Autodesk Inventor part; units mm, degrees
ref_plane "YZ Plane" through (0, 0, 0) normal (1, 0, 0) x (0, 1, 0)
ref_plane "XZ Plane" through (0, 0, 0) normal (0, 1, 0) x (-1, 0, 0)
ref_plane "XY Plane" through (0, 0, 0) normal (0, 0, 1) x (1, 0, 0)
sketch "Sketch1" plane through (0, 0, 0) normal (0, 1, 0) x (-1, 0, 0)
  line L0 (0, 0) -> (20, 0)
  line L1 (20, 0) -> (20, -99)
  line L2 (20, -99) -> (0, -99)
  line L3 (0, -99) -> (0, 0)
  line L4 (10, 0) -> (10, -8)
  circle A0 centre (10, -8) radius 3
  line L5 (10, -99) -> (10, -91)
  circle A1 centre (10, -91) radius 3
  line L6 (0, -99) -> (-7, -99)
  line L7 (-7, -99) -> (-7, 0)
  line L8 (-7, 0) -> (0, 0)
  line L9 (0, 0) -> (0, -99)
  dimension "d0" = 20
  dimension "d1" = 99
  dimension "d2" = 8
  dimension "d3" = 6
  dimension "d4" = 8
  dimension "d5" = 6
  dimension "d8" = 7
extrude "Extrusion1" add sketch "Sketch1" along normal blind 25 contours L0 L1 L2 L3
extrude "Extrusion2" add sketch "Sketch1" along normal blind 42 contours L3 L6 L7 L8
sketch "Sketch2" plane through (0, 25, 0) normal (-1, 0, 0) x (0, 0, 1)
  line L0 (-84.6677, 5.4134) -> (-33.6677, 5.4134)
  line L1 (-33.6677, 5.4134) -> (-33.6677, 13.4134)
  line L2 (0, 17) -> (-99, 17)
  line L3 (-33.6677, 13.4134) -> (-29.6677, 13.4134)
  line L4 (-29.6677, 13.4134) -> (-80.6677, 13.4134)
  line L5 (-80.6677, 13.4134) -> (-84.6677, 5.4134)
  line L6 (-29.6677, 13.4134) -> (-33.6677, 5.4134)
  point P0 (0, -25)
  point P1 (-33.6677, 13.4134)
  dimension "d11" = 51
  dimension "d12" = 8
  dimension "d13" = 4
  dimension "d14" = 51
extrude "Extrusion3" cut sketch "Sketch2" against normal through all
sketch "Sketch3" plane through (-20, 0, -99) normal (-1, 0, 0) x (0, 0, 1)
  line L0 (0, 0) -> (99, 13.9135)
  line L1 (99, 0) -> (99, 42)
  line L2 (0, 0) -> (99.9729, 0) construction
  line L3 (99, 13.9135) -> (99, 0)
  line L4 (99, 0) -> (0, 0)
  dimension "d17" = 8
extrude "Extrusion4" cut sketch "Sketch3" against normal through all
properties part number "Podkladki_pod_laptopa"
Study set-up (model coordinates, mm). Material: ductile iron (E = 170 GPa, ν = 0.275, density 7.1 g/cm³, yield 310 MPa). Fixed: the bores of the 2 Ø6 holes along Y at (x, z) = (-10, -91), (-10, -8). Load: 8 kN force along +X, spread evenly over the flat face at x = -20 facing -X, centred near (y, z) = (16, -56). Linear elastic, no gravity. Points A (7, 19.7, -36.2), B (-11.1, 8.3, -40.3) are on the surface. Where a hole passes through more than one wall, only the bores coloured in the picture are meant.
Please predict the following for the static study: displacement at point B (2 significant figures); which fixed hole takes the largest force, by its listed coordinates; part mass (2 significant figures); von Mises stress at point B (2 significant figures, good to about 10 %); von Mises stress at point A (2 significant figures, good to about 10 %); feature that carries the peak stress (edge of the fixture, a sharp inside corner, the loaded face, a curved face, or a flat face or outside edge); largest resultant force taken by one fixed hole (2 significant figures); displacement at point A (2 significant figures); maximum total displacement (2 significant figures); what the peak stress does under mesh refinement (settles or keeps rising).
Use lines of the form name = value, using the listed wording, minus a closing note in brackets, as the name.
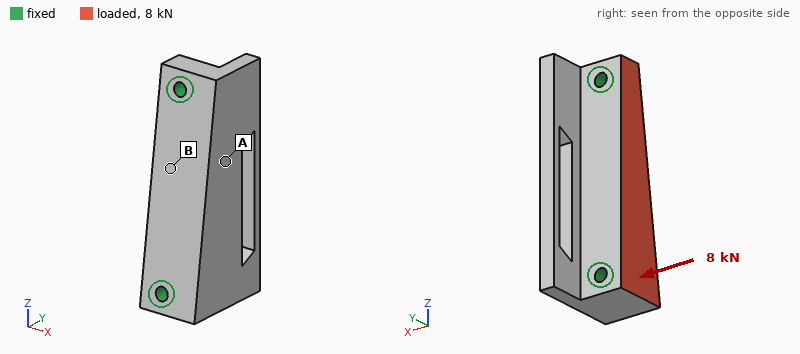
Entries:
displacement at point B = 6.7 µm
which fixed hole takes the largest force, by its listed coordinates = (-10, -91)
part mass = 400 g
von Mises stress at point B = 5.2 MPa
von Mises stress at point A = 17 MPa
feature that carries the peak stress = edge of the fixture
largest resultant force taken by one fixed hole = 4.8 kN
displacement at point A = 6.0 µm
maximum total displacement = 7.1 µm
what the peak stress does under mesh refinement = keeps rising
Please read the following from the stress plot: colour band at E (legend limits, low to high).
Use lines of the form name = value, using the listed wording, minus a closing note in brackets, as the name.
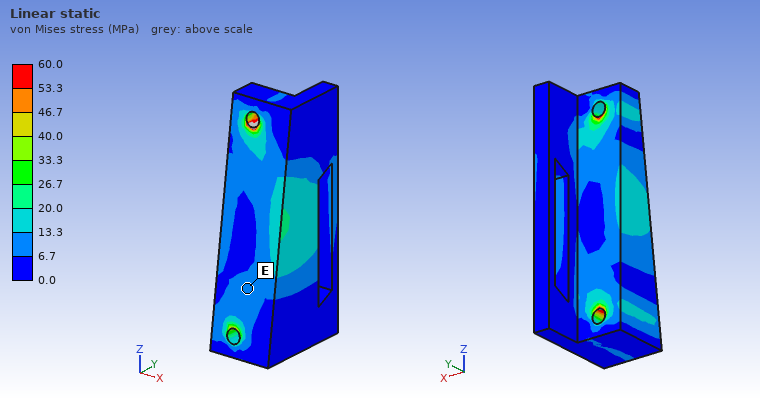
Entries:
colour band at E = 6.7 to 13.3 MPa
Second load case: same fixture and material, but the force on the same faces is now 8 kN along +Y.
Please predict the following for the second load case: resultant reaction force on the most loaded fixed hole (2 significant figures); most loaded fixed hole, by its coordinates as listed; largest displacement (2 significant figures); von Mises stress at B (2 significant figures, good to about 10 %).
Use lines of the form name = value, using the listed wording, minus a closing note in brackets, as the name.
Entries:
resultant reaction force on the most loaded fixed hole = 5.0 kN
most loaded fixed hole, by its coordinates as listed = (-10, -91)
largest displacement = 15 µm
von Mises stress at B = 21 MPa
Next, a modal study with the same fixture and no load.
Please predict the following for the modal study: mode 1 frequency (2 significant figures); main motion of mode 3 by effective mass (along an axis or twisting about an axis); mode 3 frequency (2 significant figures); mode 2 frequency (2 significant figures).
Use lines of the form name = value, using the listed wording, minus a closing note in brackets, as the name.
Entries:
mode 1 frequency = 5800 Hz
main motion of mode 3 by effective mass = along Y
mode 3 frequency = 8900 Hz
mode 2 frequency = 6600 Hz
